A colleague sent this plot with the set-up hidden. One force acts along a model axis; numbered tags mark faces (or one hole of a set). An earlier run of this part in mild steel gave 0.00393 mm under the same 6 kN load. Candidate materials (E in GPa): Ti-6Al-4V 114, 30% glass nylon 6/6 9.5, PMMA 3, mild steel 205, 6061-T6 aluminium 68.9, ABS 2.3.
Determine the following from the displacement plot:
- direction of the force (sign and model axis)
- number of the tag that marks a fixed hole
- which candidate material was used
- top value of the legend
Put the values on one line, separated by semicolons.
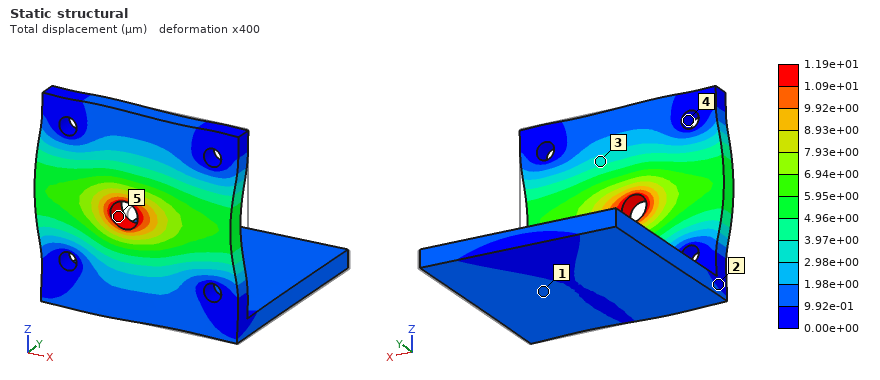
-X; 4; 6061-T6 aluminium; 1.19e+01 µm
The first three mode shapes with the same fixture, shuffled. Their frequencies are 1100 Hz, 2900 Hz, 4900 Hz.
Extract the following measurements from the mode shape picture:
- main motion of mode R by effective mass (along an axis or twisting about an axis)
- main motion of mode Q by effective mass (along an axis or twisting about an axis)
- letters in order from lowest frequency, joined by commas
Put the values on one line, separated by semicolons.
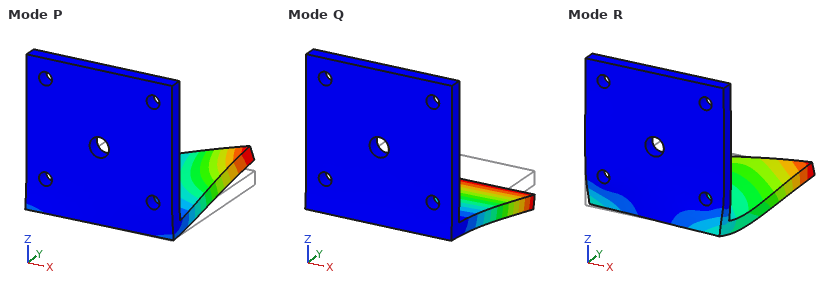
along X; along Z; Q, P, R
